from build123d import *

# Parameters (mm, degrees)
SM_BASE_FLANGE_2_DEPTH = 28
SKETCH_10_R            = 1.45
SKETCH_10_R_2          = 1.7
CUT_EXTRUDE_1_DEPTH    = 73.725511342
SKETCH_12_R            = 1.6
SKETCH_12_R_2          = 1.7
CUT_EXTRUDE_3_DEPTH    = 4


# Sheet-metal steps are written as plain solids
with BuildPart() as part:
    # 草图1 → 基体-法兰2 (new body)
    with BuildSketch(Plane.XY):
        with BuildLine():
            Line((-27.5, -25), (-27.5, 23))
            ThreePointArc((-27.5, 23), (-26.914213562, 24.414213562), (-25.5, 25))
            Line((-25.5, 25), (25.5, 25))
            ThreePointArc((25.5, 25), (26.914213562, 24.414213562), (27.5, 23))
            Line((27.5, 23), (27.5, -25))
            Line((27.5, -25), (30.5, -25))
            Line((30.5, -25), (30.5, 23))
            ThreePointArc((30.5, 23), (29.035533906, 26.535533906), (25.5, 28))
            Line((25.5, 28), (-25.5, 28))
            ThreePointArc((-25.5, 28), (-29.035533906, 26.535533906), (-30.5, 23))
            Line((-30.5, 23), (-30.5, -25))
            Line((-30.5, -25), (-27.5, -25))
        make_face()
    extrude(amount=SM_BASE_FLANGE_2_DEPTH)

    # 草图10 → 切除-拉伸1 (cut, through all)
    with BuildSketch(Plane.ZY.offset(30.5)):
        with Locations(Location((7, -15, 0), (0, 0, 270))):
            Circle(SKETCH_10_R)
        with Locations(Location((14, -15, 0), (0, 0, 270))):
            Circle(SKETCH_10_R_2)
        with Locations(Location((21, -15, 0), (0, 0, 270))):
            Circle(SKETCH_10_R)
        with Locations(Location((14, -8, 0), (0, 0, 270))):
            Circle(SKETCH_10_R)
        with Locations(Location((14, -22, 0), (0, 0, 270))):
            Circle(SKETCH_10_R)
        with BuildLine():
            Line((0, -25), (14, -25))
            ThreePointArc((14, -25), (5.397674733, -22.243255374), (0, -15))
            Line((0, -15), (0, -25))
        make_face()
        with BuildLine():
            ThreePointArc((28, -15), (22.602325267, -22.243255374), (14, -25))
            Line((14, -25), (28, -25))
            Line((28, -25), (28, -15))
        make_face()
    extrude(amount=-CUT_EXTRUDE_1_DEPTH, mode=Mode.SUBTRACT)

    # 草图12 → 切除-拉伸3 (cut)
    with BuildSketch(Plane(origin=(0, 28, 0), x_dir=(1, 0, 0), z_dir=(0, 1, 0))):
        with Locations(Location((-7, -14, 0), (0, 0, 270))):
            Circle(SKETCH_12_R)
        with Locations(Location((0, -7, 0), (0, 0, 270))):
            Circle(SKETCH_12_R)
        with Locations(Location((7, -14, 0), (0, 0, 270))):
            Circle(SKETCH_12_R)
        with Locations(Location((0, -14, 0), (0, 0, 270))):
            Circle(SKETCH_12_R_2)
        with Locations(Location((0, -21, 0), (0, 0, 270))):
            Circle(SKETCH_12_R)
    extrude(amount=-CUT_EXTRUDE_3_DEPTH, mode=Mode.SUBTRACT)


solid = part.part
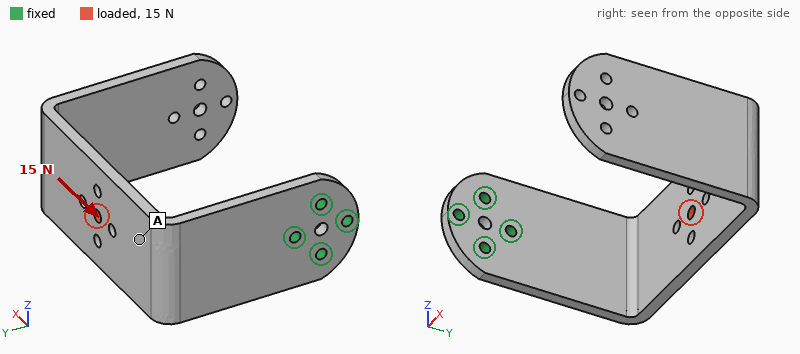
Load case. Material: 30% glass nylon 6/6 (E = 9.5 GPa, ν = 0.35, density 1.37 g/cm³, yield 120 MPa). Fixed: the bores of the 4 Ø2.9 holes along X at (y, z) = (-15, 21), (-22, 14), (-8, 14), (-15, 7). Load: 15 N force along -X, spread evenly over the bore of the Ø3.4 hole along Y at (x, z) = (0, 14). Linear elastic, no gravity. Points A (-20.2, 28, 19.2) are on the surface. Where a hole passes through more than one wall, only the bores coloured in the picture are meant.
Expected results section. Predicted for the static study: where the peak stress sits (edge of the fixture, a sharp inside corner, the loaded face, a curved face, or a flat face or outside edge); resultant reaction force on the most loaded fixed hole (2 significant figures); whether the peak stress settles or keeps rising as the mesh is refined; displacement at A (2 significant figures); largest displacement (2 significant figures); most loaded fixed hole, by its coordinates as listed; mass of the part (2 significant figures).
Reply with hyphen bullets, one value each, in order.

- edge of the fixture
- 48 N
- keeps rising
- 0.39 mm
- 0.97 mm
- (-8, 14)
- 17 g
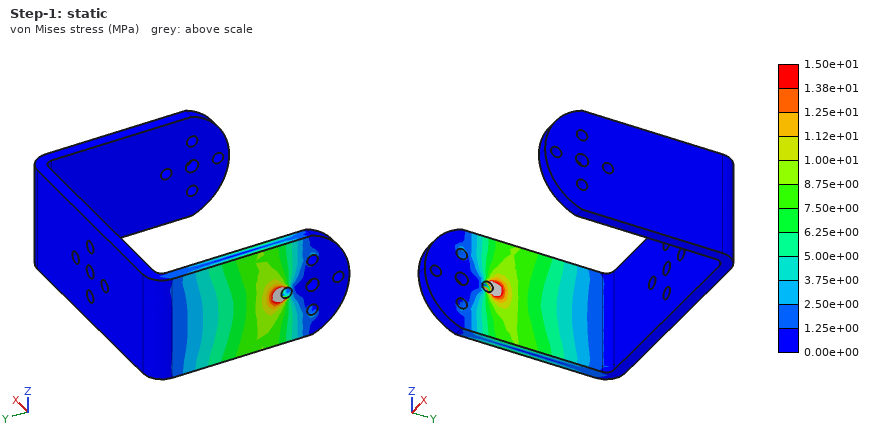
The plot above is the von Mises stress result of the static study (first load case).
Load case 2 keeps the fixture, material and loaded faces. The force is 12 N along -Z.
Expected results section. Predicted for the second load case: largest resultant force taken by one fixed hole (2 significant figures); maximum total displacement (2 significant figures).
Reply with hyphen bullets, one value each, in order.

- 21 N
- 0.85 mm
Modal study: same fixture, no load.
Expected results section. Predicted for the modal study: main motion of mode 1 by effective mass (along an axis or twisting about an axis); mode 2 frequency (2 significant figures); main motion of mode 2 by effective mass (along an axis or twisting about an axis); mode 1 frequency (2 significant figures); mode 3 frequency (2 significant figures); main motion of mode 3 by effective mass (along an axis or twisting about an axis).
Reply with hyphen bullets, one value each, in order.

- along Y
- 140 Hz
- along Z
- 100 Hz
- 270 Hz
- along X
